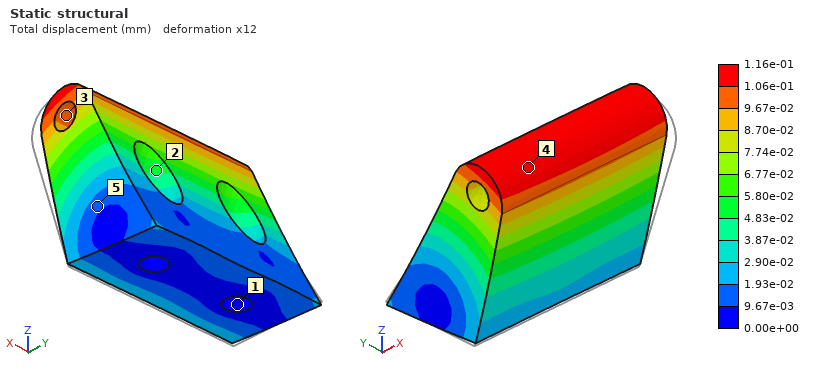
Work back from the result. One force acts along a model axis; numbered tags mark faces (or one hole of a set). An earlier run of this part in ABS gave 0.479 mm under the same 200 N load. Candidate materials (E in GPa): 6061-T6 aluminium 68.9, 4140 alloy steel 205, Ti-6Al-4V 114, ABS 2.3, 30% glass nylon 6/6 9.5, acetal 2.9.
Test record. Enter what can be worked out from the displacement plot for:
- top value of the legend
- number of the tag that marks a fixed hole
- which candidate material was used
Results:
1.16e-01 mm
1
30% glass nylon 6/6
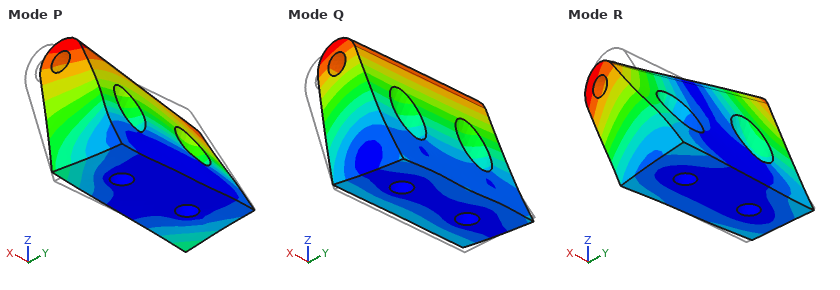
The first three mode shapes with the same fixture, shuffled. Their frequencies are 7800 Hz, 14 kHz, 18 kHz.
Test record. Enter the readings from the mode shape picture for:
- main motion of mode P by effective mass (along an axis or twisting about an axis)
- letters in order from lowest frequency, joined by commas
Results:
along X
Q, P, R
